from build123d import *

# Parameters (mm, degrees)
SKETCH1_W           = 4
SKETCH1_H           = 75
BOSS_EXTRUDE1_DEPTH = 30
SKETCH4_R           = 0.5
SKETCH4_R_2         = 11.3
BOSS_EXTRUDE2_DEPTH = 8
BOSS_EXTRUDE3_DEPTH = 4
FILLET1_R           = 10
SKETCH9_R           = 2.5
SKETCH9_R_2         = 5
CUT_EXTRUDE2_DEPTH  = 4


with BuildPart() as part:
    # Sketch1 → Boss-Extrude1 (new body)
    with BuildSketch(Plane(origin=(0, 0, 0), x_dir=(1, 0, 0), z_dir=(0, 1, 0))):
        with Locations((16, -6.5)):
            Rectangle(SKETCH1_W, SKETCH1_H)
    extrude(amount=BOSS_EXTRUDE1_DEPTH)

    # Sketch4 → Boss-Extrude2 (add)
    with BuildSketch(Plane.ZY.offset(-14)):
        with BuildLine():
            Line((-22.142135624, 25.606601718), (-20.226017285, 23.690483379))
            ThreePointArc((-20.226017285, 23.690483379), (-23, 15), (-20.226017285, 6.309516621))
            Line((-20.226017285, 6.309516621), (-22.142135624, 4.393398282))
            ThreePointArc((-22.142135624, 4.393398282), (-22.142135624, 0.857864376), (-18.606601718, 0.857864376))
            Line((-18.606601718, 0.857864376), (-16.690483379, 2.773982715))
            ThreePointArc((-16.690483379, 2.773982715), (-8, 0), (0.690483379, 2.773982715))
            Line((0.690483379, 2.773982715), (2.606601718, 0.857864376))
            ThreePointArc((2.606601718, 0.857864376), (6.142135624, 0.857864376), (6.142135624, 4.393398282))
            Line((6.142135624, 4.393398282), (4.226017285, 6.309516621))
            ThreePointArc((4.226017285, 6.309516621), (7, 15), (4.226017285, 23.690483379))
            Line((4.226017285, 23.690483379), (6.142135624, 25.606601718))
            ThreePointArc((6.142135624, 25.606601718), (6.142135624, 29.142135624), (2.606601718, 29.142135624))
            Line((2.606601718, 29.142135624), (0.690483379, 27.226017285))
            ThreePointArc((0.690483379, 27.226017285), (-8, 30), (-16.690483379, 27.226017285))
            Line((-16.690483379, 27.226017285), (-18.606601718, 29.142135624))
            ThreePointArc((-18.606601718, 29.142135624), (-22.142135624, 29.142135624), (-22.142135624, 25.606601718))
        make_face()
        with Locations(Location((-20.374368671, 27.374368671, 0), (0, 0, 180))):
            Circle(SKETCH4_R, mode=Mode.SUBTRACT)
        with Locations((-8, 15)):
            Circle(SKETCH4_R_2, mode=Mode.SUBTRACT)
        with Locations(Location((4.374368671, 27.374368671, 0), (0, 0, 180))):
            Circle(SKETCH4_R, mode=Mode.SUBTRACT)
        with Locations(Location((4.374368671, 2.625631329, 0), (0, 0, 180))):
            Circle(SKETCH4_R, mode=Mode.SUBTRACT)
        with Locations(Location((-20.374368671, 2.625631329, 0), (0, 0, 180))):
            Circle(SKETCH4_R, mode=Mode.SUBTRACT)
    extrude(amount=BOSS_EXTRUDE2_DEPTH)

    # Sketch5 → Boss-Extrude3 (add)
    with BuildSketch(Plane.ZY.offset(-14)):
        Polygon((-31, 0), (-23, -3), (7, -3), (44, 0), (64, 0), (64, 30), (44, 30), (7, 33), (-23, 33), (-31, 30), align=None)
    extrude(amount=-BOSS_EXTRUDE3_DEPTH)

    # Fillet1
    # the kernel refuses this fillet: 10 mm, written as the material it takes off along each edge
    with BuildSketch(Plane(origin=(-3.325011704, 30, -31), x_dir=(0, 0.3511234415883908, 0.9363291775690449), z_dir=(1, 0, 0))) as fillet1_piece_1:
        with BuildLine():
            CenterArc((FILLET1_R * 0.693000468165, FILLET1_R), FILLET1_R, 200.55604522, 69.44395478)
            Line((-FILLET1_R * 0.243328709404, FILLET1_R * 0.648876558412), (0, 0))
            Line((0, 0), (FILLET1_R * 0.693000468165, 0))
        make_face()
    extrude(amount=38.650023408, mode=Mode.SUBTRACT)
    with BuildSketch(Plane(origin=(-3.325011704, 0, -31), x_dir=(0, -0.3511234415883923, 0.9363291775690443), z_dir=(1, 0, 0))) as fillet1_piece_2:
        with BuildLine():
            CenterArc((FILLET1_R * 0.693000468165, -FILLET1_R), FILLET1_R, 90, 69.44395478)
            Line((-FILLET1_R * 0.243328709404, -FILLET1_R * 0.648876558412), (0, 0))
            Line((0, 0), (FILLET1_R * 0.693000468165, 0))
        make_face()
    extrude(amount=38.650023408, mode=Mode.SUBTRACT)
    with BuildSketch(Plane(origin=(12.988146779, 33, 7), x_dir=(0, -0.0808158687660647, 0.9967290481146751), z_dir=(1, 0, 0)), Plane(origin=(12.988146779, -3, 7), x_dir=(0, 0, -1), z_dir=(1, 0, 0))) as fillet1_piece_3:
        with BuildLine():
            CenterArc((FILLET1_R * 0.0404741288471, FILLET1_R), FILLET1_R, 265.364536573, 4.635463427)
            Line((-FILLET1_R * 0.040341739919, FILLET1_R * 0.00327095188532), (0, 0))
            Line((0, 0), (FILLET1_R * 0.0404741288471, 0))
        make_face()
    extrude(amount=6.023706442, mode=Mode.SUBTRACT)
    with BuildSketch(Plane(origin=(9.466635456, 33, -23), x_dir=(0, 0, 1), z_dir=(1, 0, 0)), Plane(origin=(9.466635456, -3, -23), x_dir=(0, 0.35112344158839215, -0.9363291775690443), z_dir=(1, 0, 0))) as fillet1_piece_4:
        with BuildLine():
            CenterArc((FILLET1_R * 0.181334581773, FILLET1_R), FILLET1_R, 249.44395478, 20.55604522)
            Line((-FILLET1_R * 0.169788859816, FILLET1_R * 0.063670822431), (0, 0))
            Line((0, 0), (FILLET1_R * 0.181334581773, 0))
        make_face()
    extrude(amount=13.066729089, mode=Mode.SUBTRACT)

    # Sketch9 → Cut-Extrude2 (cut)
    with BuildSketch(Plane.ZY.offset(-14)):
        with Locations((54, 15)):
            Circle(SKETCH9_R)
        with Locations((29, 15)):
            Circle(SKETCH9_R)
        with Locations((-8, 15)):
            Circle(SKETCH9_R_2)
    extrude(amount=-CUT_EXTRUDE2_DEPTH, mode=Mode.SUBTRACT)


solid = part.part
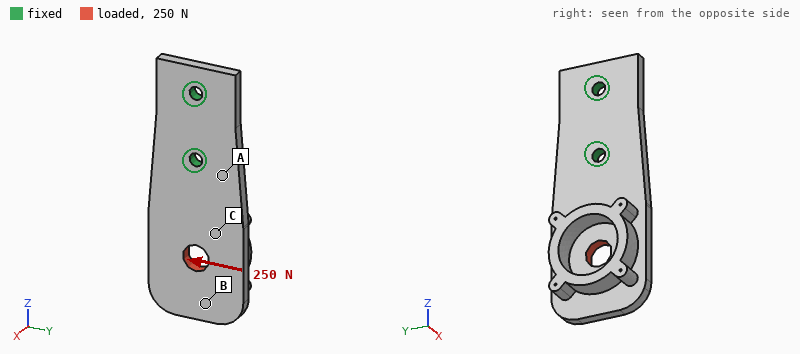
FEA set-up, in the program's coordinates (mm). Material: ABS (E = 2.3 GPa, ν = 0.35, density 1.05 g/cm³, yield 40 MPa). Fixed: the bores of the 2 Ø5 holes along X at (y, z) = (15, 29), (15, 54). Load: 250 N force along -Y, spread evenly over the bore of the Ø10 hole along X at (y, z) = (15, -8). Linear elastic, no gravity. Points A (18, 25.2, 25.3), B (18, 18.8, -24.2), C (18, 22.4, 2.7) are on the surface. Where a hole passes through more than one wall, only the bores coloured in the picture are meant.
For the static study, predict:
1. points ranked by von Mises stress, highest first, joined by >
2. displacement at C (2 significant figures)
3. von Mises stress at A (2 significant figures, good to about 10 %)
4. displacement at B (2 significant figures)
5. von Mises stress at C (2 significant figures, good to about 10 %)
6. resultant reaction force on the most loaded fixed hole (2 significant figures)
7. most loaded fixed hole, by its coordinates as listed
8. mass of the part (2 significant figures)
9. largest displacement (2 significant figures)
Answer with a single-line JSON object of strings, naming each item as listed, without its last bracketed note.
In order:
{"points ranked by von Mises stress, highest first, joined by >": "A > C > B", "displacement at C": "0.33 mm", "von Mises stress at A": "7.3 MPa", "displacement at B": "0.69 mm", "von Mises stress at C": "3.8 MPa", "resultant reaction force on the most loaded fixed hole": "540 N", "most loaded fixed hole, by its coordinates as listed": "(15, 29)", "mass of the part": "16 g", "largest displacement": "0.78 mm"}
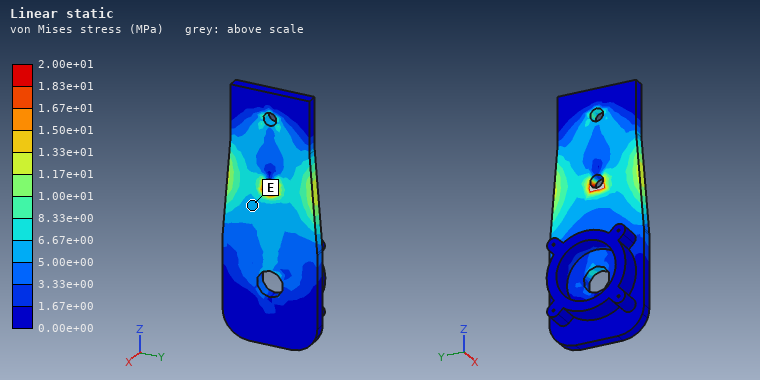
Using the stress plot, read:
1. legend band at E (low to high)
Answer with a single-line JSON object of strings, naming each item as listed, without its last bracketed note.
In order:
{"legend band at E": "5.00e+00 to 6.67e+00 MPa"}
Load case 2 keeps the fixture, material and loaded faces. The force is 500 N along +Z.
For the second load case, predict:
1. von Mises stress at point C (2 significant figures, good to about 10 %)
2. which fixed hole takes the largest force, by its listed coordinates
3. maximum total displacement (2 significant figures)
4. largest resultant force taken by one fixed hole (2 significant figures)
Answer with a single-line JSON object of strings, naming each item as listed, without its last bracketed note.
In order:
{"von Mises stress at point C": "4.6 MPa", "which fixed hole takes the largest force, by its listed coordinates": "(15, 29)", "maximum total displacement": "0.12 mm", "largest resultant force taken by one fixed hole": "390 N"}
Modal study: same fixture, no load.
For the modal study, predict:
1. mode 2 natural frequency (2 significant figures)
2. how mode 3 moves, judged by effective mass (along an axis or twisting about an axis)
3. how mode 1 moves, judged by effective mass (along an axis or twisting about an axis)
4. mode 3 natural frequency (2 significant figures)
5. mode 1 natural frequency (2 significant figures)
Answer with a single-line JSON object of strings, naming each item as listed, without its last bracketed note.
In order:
{"mode 2 natural frequency": "750 Hz", "how mode 3 moves, judged by effective mass": "along Y", "how mode 1 moves, judged by effective mass": "along X", "mode 3 natural frequency": "1100 Hz", "mode 1 natural frequency": "230 Hz"}
